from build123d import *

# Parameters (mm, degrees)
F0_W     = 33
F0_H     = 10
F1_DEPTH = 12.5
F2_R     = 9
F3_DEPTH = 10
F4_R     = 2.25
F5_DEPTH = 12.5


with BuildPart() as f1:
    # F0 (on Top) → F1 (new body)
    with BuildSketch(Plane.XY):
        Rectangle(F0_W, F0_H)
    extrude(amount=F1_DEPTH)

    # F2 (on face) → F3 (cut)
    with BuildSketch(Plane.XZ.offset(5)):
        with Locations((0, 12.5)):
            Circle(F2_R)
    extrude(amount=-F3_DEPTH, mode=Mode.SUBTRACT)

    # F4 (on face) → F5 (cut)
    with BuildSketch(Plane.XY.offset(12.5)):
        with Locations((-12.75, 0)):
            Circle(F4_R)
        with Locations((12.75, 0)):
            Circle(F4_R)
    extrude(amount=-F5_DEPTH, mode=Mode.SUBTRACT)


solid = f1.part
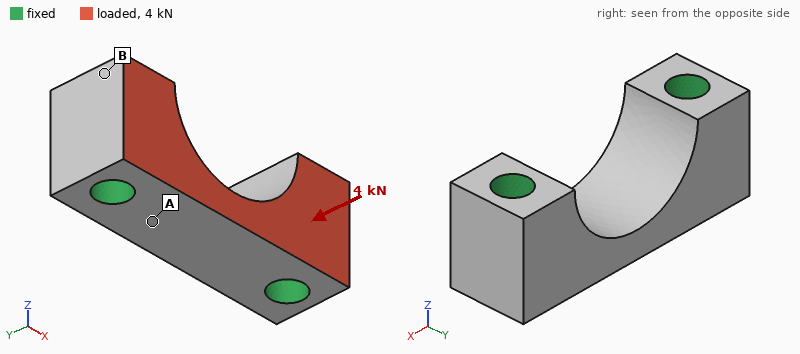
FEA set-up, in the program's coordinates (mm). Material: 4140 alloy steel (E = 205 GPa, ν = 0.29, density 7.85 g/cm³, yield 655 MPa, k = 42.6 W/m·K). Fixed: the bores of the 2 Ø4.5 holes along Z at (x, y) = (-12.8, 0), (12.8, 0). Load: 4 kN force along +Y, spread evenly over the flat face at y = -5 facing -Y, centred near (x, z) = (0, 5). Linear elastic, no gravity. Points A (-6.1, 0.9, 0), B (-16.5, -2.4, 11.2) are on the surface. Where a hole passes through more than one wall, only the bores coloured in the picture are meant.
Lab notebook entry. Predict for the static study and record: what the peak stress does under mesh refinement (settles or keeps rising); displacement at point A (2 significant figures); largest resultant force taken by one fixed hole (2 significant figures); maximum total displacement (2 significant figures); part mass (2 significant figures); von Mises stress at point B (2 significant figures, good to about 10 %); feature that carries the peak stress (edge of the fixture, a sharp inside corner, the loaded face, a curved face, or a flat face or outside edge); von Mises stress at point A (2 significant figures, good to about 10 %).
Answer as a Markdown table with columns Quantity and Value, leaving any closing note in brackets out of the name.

| Quantity | Value |
|---|---|
| what the peak stress does under mesh refinement | keeps rising |
| displacement at point A | 1.3 µm |
| largest resultant force taken by one fixed hole | 2.0 kN |
| maximum total displacement | 2.4 µm |
| part mass | 19 g |
| von Mises stress at point B | 8.6 MPa |
| feature that carries the peak stress | edge of the fixture |
| von Mises stress at point A | 22 MPa |
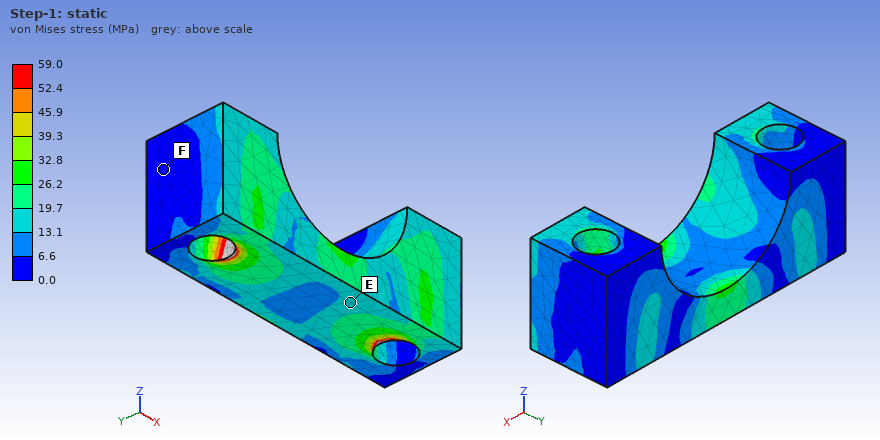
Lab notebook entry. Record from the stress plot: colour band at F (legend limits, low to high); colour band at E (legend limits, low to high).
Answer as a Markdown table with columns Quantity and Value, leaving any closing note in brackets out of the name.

| Quantity | Value |
|---|---|
| colour band at F | 0.0 to 6.6 MPa |
| colour band at E | 13.1 to 19.7 MPa |
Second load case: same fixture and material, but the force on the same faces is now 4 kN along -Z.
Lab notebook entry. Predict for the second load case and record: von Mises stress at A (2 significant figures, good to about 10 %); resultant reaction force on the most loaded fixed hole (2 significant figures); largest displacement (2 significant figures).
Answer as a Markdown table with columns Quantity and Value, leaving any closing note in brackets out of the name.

| Quantity | Value |
|---|---|
| von Mises stress at A | 28 MPa |
| resultant reaction force on the most loaded fixed hole | 2.0 kN |
| largest displacement | 5.1 µm |
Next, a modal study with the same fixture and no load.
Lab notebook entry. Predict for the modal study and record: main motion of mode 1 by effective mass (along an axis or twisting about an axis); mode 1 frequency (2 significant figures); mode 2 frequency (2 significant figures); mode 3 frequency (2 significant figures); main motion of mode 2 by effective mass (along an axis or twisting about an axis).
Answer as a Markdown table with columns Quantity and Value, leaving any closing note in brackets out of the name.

| Quantity | Value |
|---|---|
| main motion of mode 1 by effective mass | along Y |
| mode 1 frequency | 56 kHz |
| mode 2 frequency | 63 kHz |
| mode 3 frequency | 86 kHz |
| main motion of mode 2 by effective mass | along Z |
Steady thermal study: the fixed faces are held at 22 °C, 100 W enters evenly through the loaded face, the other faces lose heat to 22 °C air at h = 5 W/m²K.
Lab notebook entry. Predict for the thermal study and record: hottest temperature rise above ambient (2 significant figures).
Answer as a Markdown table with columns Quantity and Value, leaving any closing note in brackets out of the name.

| Quantity | Value |
|---|---|
| hottest temperature rise above ambient | 71 K |
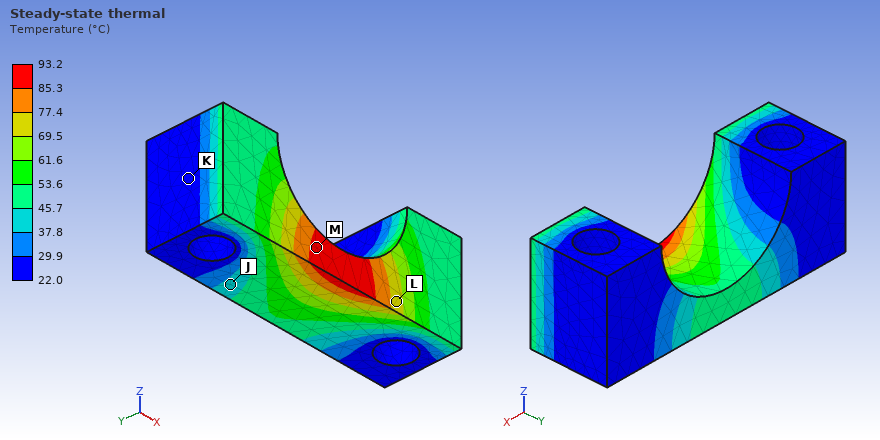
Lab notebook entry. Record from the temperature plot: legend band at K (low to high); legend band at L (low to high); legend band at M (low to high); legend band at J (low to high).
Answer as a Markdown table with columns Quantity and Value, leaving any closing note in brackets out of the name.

| Quantity | Value |
|---|---|
| legend band at K | 22.0 to 29.9 °C |
| legend band at L | 69.5 to 77.4 °C |
| legend band at M | 85.3 to 93.2 °C |
| legend band at J | 37.8 to 45.7 °C |
